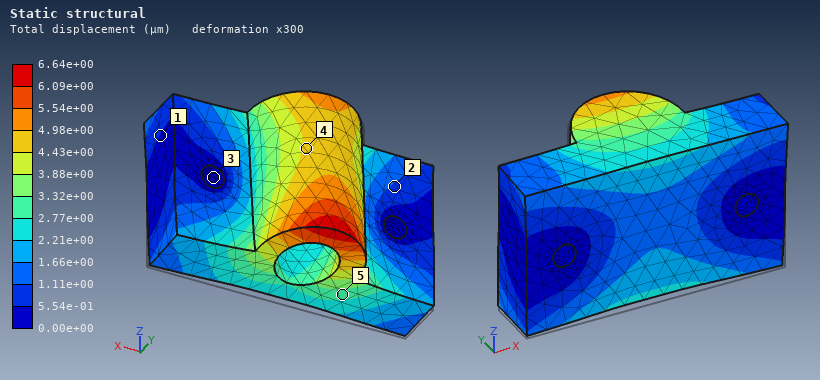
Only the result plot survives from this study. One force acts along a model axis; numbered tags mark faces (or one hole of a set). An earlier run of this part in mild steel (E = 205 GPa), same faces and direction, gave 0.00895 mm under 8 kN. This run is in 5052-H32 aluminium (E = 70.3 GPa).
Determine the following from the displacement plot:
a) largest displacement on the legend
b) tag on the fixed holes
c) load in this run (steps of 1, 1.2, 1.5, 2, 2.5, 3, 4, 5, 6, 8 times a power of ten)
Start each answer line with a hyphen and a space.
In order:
- 6.64e+00 µm
- 3
- 2 kN
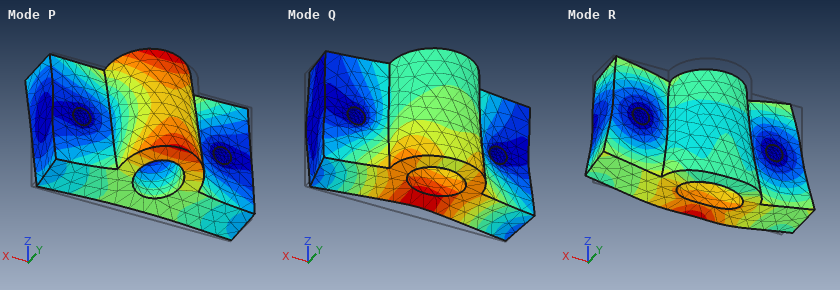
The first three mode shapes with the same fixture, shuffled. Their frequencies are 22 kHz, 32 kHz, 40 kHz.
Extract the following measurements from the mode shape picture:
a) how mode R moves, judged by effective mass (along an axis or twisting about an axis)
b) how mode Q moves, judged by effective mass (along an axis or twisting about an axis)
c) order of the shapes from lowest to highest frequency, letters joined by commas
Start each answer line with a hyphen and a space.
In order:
- along Z
- along Y
- P, Q, R
